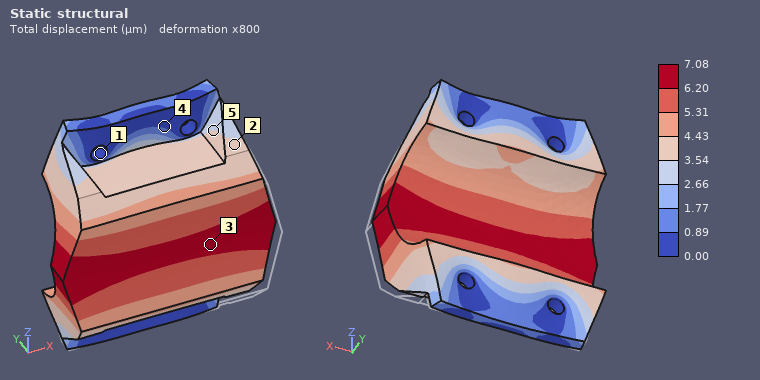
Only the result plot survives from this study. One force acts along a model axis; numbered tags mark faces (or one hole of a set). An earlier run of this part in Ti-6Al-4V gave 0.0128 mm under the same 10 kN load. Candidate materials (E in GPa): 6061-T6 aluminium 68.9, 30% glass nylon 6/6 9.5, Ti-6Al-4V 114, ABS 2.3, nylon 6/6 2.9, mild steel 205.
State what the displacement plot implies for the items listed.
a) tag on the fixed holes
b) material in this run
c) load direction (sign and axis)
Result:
1
mild steel
+Y
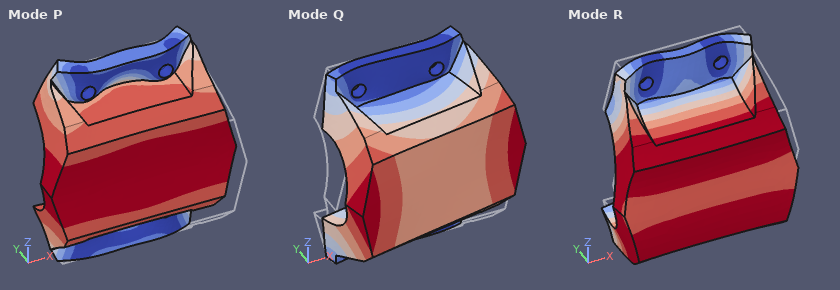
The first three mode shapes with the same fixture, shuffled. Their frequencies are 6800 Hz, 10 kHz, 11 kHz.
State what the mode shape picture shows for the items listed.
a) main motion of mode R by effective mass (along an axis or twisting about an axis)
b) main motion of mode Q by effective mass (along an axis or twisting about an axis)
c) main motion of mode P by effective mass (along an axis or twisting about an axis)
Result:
along Z
along X
along Y
